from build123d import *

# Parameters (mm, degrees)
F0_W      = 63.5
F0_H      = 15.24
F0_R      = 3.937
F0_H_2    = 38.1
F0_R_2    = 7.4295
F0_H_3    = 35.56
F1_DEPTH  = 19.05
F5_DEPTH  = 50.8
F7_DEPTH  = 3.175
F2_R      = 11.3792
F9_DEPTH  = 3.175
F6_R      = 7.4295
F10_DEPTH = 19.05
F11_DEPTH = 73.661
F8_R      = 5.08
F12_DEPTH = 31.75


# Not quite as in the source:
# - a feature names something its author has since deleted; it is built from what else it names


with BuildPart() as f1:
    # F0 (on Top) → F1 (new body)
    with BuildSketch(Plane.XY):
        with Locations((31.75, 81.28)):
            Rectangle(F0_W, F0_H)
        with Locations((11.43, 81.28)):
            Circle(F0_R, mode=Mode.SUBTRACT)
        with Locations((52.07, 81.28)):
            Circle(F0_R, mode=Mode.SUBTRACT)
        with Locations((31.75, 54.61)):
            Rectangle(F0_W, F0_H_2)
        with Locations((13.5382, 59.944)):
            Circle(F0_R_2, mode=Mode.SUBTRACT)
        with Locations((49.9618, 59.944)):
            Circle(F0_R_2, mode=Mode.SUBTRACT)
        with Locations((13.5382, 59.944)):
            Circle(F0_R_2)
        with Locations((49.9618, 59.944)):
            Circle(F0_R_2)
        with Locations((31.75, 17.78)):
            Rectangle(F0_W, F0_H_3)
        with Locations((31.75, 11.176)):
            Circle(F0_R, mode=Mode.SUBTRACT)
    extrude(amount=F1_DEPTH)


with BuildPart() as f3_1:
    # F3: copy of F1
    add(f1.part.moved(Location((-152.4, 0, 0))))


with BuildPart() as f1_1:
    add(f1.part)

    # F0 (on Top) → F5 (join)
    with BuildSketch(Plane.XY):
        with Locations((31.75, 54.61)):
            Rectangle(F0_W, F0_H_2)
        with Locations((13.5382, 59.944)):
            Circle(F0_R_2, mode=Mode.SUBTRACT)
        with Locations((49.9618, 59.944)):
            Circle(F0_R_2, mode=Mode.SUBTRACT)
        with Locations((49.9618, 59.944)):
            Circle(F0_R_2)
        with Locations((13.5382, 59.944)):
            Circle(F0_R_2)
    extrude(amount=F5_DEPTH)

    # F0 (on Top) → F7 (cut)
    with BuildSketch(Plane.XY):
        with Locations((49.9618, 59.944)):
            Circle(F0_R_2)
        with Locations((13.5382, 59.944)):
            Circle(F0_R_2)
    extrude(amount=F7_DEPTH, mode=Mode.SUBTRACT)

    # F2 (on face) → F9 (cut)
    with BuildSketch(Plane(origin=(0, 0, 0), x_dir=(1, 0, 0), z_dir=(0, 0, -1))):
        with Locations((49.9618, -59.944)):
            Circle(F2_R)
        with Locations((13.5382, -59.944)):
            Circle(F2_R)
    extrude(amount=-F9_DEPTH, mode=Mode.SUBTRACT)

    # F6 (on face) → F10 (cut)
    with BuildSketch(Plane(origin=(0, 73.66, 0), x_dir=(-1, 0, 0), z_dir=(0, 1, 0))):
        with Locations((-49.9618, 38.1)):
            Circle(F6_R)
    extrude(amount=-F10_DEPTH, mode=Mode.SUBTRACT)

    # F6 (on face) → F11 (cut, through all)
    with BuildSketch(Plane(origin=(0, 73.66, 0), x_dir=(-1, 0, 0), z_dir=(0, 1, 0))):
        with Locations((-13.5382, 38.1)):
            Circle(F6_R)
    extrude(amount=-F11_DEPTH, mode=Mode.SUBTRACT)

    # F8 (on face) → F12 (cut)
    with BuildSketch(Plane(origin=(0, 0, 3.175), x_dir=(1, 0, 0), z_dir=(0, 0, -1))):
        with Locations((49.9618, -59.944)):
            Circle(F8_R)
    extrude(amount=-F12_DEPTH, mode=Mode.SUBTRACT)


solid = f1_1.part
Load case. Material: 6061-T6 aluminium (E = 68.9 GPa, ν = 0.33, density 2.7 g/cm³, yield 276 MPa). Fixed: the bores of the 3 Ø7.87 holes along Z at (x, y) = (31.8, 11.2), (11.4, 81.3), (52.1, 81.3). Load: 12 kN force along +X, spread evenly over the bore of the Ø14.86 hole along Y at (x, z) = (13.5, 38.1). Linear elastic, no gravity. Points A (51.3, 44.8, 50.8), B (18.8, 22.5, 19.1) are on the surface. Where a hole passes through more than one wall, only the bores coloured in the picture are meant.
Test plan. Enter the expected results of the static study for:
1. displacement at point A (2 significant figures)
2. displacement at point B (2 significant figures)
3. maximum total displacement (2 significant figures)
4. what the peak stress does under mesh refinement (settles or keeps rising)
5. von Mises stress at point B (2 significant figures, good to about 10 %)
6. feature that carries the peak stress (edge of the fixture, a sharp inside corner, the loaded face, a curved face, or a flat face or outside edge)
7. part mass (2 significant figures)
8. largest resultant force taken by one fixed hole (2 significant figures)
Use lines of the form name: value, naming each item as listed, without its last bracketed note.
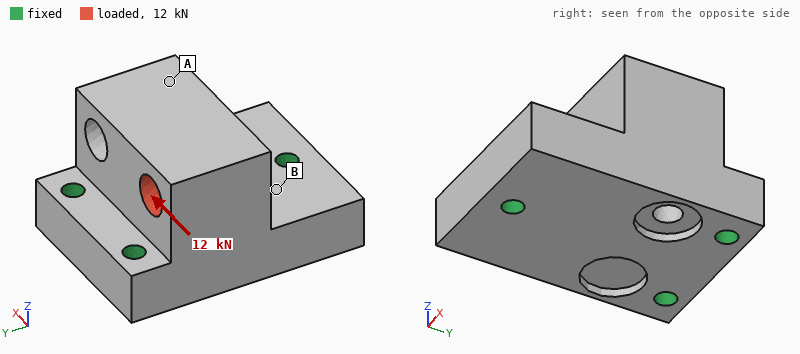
displacement at point A: 34 µm
displacement at point B: 8.0 µm
maximum total displacement: 42 µm
what the peak stress does under mesh refinement: keeps rising
von Mises stress at point B: 15 MPa
feature that carries the peak stress: edge of the fixture
part mass: 450 g
largest resultant force taken by one fixed hole: 8.0 kN
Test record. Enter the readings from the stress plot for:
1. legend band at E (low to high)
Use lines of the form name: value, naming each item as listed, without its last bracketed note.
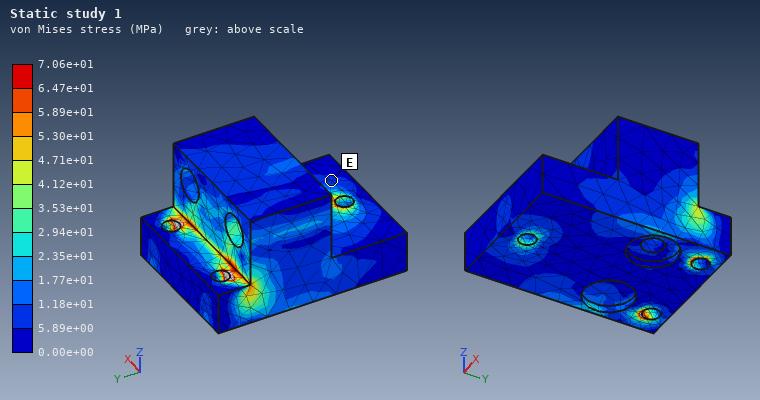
legend band at E: 5.89e+00 to 1.18e+01 MPa
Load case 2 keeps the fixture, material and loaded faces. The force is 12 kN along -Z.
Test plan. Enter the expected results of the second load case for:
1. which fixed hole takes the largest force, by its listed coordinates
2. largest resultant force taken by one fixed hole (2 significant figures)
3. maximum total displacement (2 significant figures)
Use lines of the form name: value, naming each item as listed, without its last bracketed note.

which fixed hole takes the largest force, by its listed coordinates: (11.4, 81.3)
largest resultant force taken by one fixed hole: 7.9 kN
maximum total displacement: 34 µm
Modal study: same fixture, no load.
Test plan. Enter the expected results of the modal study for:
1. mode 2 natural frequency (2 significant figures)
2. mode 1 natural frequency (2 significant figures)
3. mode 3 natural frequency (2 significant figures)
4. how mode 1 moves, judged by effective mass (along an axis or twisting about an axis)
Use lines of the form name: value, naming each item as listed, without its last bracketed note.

mode 2 natural frequency: 7800 Hz
mode 1 natural frequency: 7200 Hz
mode 3 natural frequency: 13 kHz
how mode 1 moves, judged by effective mass: along X
